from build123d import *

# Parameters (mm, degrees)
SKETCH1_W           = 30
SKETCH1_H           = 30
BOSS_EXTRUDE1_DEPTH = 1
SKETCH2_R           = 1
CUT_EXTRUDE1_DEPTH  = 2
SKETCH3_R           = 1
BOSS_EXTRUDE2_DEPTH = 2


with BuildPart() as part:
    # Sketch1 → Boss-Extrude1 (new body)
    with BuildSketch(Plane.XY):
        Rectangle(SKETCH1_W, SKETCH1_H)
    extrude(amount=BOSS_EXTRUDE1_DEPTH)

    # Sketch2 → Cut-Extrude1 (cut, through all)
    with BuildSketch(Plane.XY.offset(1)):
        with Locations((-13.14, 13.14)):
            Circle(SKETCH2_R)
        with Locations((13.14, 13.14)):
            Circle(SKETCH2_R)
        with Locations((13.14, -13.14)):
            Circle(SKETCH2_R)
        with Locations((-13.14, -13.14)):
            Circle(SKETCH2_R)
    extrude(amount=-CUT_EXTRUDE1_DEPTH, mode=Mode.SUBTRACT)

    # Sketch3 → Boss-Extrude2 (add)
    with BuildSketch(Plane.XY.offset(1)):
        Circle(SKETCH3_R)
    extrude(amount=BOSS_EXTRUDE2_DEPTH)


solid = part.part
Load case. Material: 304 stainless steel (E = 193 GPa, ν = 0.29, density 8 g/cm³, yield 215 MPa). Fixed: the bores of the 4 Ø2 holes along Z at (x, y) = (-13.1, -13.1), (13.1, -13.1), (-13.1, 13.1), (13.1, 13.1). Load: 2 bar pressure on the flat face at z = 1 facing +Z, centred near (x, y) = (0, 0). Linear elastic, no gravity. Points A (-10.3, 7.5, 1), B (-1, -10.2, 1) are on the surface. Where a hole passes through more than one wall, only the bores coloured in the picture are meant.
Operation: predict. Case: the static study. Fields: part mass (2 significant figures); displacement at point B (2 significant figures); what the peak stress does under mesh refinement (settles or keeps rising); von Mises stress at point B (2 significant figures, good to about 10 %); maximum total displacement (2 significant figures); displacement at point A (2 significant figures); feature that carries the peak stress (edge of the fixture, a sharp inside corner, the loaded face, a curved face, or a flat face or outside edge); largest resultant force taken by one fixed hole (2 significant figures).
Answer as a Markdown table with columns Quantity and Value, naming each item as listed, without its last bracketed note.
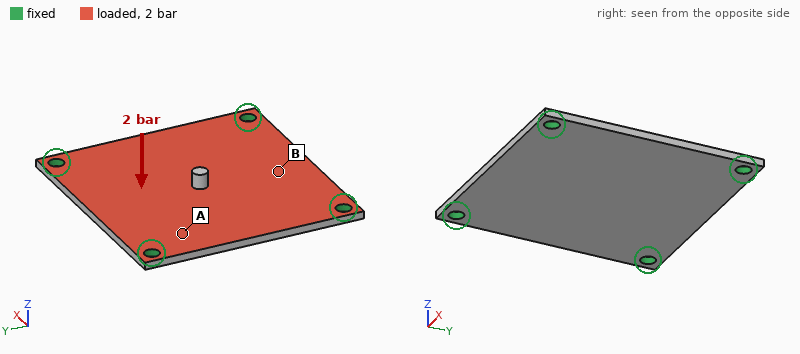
| Quantity | Value |
|---|---|
| part mass | 7.1 g |
| displacement at point B | 25 µm |
| what the peak stress does under mesh refinement | keeps rising |
| von Mises stress at point B | 41 MPa |
| maximum total displacement | 38 µm |
| displacement at point A | 14 µm |
| feature that carries the peak stress | edge of the fixture |
| largest resultant force taken by one fixed hole | 44 N |
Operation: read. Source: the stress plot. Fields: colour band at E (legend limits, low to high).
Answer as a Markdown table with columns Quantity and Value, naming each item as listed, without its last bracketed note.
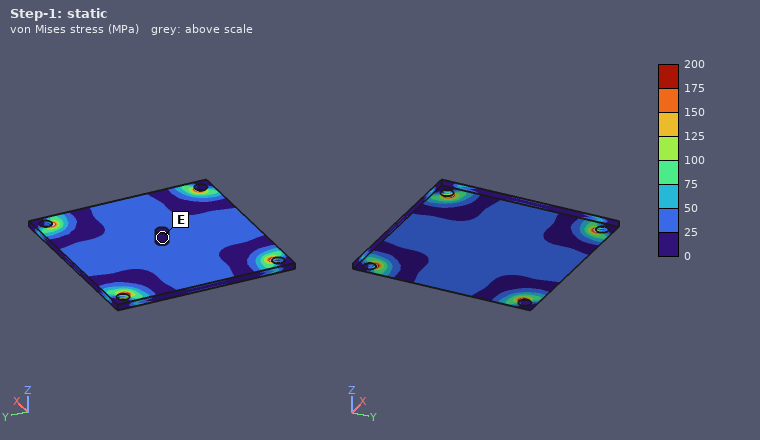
| Quantity | Value |
|---|---|
| colour band at E | 0 to 25 MPa |
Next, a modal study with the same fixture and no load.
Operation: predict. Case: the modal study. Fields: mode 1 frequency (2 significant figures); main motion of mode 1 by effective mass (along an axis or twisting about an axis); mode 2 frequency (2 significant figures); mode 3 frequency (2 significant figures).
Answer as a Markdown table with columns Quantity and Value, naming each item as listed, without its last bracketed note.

| Quantity | Value |
|---|---|
| mode 1 frequency | 4900 Hz |
| main motion of mode 1 by effective mass | along Z |
| mode 2 frequency | 8600 Hz |
| mode 3 frequency | 8600 Hz |
